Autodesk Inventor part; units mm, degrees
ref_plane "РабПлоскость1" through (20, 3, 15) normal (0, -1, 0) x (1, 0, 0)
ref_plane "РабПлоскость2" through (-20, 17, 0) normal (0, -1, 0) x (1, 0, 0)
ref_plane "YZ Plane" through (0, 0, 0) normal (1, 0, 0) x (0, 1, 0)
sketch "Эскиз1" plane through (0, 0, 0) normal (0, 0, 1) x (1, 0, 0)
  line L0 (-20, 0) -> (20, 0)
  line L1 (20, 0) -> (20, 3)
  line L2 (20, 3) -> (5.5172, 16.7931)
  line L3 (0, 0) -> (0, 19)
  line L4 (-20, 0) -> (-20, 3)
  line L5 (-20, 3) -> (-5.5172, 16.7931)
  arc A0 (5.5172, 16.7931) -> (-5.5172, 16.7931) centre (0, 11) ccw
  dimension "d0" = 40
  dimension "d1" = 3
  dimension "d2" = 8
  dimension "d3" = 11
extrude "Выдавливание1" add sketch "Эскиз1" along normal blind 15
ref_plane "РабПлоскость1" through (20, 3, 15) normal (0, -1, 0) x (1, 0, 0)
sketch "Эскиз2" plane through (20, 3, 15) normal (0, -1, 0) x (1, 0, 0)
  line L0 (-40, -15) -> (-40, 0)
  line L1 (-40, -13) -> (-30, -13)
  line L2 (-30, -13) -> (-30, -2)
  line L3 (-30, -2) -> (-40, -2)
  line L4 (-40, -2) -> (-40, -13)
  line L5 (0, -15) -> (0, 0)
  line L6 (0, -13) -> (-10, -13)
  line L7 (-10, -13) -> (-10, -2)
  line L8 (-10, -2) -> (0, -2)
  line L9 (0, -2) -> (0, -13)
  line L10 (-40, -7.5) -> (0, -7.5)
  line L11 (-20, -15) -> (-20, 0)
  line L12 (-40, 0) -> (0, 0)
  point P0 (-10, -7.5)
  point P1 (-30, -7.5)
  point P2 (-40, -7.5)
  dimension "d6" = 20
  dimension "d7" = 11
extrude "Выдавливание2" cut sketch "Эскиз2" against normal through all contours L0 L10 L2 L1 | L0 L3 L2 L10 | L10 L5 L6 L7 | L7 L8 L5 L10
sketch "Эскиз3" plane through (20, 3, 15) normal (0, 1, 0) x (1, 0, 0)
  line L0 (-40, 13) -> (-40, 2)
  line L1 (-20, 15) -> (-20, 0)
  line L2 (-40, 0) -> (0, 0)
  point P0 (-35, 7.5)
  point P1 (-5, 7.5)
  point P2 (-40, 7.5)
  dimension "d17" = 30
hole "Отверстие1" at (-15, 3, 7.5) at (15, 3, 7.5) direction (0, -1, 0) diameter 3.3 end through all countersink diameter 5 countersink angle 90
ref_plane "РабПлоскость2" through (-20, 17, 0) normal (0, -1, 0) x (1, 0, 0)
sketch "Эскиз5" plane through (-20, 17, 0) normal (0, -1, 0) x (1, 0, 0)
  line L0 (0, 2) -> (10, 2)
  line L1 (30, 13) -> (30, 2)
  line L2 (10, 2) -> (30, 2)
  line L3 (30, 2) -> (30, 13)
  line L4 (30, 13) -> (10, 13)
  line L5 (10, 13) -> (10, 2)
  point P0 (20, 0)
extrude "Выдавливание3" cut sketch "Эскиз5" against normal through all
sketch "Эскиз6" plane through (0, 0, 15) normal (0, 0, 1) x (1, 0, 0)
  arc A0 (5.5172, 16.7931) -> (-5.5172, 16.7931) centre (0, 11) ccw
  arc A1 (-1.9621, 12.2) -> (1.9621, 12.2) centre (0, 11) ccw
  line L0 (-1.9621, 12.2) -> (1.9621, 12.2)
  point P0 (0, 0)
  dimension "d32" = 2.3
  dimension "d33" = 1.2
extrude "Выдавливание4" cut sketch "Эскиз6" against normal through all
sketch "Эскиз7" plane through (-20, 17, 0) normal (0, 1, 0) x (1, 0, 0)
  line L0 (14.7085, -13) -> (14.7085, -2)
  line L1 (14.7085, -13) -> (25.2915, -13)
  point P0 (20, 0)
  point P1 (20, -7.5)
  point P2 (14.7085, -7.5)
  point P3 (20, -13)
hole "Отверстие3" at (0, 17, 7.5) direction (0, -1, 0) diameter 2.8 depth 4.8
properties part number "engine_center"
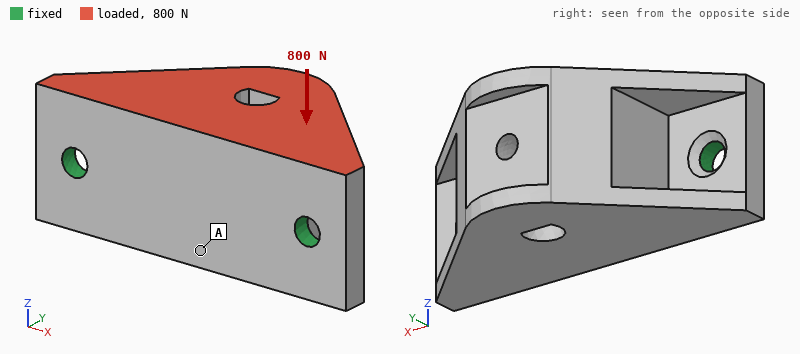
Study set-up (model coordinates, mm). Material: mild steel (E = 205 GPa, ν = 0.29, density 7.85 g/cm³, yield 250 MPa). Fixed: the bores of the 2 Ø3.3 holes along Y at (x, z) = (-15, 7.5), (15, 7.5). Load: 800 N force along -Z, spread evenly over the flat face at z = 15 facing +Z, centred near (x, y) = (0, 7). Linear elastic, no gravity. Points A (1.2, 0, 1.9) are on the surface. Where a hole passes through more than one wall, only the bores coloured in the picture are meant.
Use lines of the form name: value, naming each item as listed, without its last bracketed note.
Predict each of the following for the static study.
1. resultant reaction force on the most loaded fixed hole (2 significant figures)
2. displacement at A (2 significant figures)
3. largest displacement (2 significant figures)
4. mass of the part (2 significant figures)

resultant reaction force on the most loaded fixed hole: 400 N
displacement at A: 4.9 µm
largest displacement: 19 µm
mass of the part: 46 g
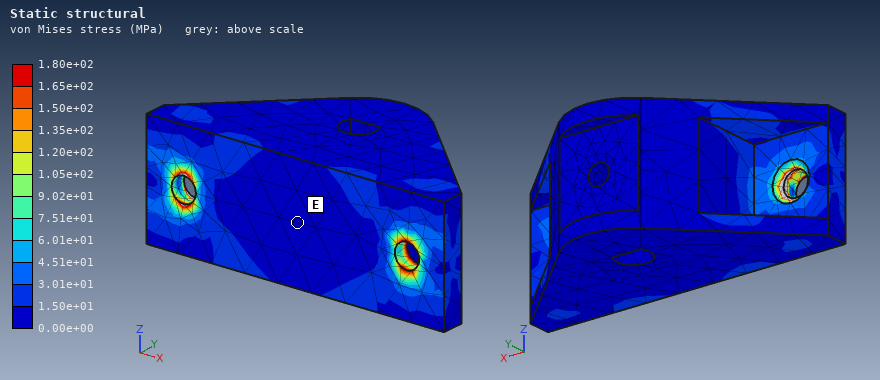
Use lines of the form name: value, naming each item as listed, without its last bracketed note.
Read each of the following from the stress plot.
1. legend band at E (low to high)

legend band at E: 0.00e+00 to 1.50e+01 MPa
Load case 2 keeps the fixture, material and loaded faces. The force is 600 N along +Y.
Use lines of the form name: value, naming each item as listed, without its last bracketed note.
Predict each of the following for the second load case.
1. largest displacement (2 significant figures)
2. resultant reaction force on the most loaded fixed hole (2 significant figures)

largest displacement: 16 µm
resultant reaction force on the most loaded fixed hole: 330 N
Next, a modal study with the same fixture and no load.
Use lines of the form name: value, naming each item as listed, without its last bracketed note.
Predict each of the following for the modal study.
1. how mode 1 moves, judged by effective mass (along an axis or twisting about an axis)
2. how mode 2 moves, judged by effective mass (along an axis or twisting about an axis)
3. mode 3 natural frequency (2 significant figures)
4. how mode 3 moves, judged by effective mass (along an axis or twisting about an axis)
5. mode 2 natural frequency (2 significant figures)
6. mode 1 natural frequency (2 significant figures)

how mode 1 moves, judged by effective mass: along Z
how mode 2 moves, judged by effective mass: along Y
mode 3 natural frequency: 21 kHz
how mode 3 moves, judged by effective mass: along X
mode 2 natural frequency: 16 kHz
mode 1 natural frequency: 6000 Hz
